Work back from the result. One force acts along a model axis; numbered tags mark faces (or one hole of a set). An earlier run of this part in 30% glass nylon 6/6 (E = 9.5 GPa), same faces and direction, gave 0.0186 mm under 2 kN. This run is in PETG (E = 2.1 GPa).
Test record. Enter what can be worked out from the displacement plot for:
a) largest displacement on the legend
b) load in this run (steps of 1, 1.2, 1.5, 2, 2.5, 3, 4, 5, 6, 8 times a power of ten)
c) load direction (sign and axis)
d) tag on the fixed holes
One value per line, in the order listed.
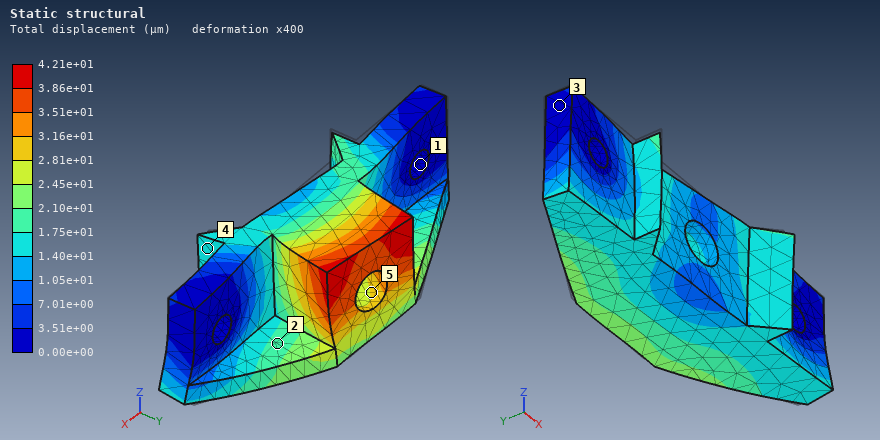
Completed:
4.21e+01 µm
1 kN
+X
1
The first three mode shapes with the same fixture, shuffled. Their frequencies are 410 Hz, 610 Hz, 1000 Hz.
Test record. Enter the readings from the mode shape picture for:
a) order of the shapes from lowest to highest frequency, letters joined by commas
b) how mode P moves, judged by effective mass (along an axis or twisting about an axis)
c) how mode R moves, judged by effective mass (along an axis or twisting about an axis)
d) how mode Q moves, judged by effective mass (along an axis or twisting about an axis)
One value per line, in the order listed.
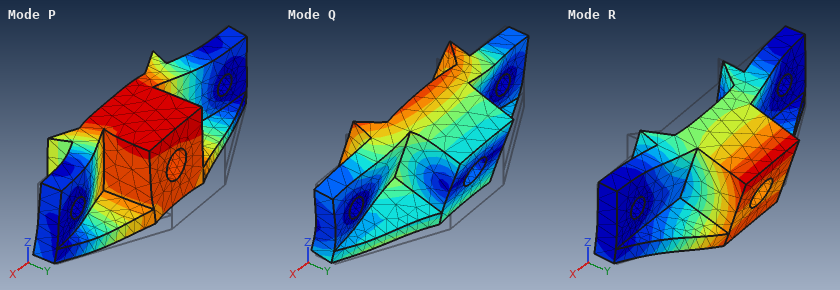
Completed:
R, P, Q
along Y
along Z
along Z
